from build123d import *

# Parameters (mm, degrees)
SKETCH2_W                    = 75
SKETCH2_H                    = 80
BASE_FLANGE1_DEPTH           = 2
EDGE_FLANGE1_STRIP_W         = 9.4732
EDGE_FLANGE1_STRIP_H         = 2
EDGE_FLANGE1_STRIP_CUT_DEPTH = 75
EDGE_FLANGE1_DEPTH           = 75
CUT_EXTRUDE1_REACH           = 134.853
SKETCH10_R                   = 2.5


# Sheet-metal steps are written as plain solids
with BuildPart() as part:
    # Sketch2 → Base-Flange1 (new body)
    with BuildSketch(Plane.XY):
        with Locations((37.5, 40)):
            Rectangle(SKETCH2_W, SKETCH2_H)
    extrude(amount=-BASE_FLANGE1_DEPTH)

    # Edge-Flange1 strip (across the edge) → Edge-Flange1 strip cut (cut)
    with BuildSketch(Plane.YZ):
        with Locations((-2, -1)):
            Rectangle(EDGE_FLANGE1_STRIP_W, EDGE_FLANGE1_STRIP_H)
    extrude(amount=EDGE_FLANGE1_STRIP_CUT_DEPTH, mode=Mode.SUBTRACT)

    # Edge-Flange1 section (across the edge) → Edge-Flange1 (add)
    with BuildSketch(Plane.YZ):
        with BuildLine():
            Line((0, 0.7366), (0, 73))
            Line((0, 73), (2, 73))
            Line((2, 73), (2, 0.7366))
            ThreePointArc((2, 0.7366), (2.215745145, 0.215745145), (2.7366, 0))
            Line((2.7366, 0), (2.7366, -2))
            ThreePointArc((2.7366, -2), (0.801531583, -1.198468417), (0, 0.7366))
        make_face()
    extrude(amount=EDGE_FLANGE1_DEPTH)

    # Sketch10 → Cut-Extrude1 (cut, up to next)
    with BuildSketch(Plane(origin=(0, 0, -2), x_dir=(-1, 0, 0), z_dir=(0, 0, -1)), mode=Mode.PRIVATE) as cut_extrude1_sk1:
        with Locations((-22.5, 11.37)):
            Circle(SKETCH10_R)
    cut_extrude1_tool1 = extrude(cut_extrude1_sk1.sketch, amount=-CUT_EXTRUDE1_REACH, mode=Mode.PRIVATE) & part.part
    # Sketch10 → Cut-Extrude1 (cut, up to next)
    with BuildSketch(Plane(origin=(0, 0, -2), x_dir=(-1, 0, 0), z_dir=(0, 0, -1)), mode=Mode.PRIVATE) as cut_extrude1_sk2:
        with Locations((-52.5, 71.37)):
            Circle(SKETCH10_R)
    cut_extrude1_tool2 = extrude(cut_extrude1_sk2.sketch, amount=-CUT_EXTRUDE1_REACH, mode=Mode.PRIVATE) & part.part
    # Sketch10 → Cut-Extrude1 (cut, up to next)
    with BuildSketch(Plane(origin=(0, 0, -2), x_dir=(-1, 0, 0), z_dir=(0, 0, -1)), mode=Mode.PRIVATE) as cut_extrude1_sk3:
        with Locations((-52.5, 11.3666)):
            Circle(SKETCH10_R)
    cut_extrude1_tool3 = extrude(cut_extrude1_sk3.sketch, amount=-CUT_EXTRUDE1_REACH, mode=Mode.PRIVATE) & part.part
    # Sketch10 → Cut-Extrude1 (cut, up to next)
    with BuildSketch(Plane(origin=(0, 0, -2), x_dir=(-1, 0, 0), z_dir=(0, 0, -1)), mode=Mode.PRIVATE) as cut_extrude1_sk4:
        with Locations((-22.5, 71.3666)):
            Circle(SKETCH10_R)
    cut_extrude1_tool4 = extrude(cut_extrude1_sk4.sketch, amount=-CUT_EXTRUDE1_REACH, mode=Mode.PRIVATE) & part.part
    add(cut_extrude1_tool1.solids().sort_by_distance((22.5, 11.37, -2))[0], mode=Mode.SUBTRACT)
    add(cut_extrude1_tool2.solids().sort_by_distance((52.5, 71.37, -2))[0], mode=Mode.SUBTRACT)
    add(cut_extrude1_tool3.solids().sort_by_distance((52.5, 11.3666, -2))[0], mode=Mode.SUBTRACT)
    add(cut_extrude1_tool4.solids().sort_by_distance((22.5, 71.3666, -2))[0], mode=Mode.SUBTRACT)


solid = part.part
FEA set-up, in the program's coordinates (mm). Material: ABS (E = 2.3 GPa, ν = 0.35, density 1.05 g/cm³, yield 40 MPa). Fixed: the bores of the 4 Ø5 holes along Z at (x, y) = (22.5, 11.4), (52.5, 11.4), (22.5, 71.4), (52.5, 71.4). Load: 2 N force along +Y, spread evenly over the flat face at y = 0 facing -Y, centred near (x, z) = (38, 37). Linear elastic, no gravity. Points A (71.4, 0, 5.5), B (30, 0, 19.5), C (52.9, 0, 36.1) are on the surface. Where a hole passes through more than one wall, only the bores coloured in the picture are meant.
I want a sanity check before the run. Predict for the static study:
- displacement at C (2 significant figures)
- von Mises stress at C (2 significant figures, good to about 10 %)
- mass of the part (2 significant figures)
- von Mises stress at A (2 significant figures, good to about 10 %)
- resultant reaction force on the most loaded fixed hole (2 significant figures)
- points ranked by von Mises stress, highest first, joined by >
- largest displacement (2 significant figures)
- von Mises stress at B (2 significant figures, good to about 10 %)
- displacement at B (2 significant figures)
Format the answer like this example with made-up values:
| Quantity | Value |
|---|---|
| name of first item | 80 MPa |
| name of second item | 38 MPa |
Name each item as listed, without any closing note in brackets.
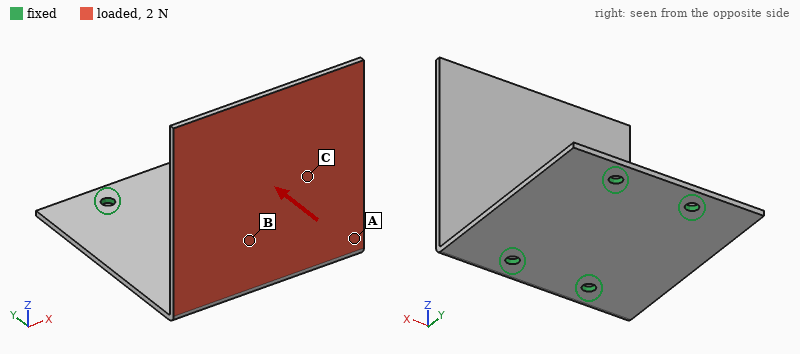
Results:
| Quantity | Value |
|---|---|
| displacement at C | 0.52 mm |
| von Mises stress at C | 0.35 MPa |
| mass of the part | 24 g |
| von Mises stress at A | 1.1 MPa |
| resultant reaction force on the most loaded fixed hole | 0.89 N |
| points ranked by von Mises stress, highest first, joined by > | A > B > C |
| largest displacement | 1.3 mm |
| von Mises stress at B | 0.70 MPa |
| displacement at B | 0.24 mm |
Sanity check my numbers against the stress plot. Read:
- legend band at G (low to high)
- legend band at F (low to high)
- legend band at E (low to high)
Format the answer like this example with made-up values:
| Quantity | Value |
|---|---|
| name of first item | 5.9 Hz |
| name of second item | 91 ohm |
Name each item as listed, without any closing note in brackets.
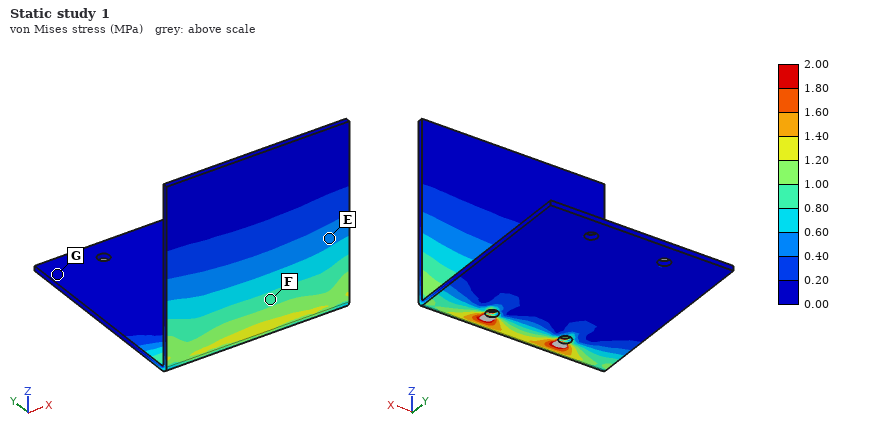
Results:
| Quantity | Value |
|---|---|
| legend band at G | 0.00 to 0.20 MPa |
| legend band at F | 0.80 to 1.00 MPa |
| legend band at E | 0.40 to 0.60 MPa |
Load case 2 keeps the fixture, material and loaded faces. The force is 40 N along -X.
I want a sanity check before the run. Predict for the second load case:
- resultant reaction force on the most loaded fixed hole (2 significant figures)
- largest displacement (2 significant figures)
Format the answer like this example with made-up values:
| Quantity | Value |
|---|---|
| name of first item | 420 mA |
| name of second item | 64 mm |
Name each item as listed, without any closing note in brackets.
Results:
| Quantity | Value |
|---|---|
| resultant reaction force on the most loaded fixed hole | 50 N |
| largest displacement | 1.2 mm |
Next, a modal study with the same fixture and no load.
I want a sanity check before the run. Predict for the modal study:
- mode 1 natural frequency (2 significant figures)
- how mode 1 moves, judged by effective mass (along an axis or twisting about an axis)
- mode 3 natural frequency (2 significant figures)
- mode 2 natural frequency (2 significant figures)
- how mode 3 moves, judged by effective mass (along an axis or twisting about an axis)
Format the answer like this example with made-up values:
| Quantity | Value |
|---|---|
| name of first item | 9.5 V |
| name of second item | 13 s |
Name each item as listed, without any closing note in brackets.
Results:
| Quantity | Value |
|---|---|
| mode 1 natural frequency | 73 Hz |
| how mode 1 moves, judged by effective mass | along Y |
| mode 3 natural frequency | 340 Hz |
| mode 2 natural frequency | 190 Hz |
| how mode 3 moves, judged by effective mass | along X |
